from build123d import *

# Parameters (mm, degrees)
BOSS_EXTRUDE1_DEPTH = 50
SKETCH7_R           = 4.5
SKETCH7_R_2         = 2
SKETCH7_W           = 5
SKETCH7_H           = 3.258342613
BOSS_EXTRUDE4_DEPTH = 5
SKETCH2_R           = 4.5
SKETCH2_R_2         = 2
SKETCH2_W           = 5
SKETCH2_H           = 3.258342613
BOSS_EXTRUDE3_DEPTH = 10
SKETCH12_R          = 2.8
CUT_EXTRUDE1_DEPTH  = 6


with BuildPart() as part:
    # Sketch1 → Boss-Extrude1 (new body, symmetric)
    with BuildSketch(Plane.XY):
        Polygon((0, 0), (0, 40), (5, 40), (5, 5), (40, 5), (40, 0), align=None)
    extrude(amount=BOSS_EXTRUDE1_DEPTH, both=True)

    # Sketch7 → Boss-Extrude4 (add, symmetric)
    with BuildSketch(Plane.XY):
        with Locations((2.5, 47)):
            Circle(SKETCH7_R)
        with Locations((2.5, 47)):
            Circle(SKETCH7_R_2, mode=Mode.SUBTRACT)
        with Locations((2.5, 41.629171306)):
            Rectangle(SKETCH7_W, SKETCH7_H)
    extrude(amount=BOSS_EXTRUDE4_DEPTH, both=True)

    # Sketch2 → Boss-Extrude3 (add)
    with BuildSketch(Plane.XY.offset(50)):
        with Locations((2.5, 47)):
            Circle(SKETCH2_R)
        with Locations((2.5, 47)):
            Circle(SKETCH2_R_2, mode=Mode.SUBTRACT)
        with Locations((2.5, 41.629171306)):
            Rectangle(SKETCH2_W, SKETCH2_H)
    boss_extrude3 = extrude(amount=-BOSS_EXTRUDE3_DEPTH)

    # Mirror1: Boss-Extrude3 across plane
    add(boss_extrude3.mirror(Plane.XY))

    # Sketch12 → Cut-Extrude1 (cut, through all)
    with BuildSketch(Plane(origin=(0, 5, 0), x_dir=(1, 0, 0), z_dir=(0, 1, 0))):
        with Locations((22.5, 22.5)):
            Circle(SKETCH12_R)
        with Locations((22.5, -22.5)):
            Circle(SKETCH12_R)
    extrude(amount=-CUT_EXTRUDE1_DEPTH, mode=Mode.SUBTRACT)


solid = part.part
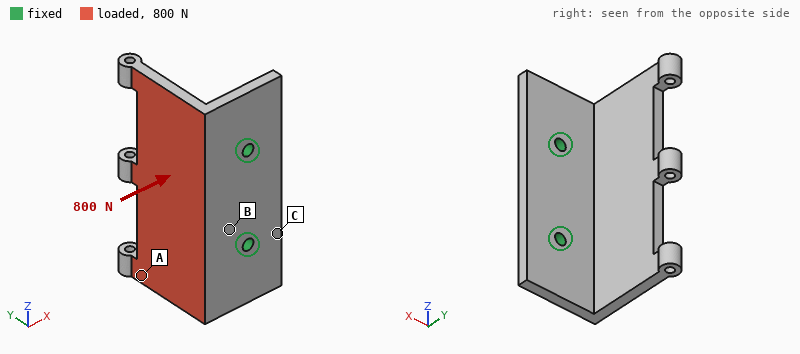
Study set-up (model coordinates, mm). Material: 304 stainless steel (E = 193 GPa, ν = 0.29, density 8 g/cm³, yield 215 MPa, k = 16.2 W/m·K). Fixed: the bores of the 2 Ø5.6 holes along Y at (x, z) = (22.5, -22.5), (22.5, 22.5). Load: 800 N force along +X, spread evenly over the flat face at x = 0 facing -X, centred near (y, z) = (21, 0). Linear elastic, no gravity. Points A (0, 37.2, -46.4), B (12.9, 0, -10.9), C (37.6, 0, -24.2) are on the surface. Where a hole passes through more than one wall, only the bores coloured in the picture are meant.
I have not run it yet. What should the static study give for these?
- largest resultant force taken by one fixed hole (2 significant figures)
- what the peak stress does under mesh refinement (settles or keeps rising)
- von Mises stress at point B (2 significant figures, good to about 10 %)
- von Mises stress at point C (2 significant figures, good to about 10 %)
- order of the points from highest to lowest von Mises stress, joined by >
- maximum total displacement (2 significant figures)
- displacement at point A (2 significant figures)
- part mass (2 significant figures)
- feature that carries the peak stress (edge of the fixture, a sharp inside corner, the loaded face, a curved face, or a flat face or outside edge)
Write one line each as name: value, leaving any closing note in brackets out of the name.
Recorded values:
largest resultant force taken by one fixed hole: 400 N
what the peak stress does under mesh refinement: keeps rising
von Mises stress at point B: 31 MPa
von Mises stress at point C: 12 MPa
order of the points from highest to lowest von Mises stress, joined by >: B > C > A
maximum total displacement: 0.11 mm
displacement at point A: 0.077 mm
part mass: 310 g
feature that carries the peak stress: edge of the fixture
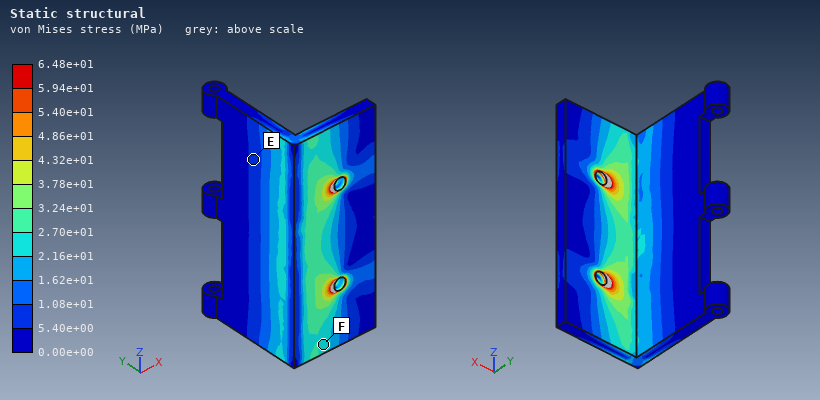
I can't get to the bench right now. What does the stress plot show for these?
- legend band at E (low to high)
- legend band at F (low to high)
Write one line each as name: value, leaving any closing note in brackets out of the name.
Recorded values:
legend band at E: 5.40e+00 to 1.08e+01 MPa
legend band at F: 2.16e+01 to 2.70e+01 MPa
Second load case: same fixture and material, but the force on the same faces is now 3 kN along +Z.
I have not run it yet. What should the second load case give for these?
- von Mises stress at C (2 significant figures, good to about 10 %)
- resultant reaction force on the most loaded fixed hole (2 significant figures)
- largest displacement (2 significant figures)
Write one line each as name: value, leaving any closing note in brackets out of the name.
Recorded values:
von Mises stress at C: 19 MPa
resultant reaction force on the most loaded fixed hole: 2.3 kN
largest displacement: 72 µm
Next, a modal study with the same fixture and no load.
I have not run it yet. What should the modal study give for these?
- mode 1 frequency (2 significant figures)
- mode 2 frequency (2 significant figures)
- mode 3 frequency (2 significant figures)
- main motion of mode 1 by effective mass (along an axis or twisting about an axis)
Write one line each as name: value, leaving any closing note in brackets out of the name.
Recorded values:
mode 1 frequency: 1200 Hz
mode 2 frequency: 1800 Hz
mode 3 frequency: 2900 Hz
main motion of mode 1 by effective mass: along X
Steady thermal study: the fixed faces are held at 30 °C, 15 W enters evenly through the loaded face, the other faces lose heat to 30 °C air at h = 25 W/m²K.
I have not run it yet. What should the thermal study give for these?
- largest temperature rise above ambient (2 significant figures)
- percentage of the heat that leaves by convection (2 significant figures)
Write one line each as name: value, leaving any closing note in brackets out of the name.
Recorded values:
largest temperature rise above ambient: 43 K
percentage of the heat that leaves by convection: 53 %
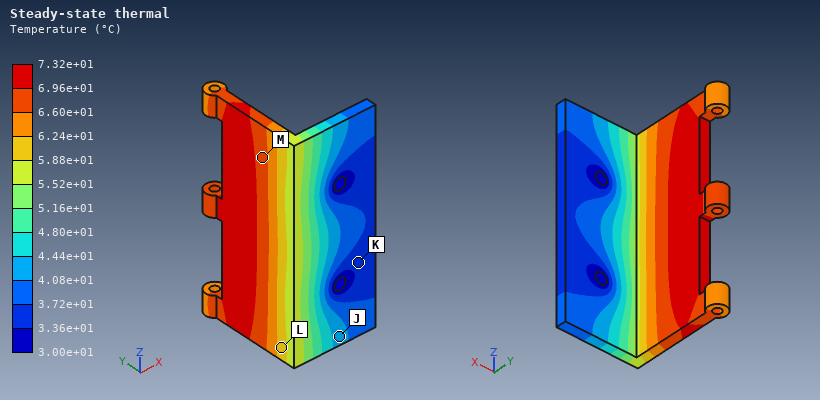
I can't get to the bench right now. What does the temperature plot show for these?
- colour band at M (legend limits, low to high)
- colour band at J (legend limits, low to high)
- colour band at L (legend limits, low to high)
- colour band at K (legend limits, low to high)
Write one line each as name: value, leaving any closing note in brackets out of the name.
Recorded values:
colour band at M: 6.60e+01 to 6.96e+01 °C
colour band at J: 4.08e+01 to 4.44e+01 °C
colour band at L: 5.88e+01 to 6.24e+01 °C
colour band at K: 3.36e+01 to 3.72e+01 °C
